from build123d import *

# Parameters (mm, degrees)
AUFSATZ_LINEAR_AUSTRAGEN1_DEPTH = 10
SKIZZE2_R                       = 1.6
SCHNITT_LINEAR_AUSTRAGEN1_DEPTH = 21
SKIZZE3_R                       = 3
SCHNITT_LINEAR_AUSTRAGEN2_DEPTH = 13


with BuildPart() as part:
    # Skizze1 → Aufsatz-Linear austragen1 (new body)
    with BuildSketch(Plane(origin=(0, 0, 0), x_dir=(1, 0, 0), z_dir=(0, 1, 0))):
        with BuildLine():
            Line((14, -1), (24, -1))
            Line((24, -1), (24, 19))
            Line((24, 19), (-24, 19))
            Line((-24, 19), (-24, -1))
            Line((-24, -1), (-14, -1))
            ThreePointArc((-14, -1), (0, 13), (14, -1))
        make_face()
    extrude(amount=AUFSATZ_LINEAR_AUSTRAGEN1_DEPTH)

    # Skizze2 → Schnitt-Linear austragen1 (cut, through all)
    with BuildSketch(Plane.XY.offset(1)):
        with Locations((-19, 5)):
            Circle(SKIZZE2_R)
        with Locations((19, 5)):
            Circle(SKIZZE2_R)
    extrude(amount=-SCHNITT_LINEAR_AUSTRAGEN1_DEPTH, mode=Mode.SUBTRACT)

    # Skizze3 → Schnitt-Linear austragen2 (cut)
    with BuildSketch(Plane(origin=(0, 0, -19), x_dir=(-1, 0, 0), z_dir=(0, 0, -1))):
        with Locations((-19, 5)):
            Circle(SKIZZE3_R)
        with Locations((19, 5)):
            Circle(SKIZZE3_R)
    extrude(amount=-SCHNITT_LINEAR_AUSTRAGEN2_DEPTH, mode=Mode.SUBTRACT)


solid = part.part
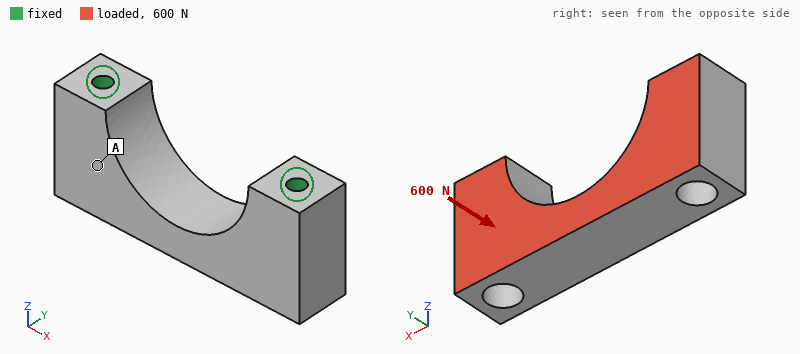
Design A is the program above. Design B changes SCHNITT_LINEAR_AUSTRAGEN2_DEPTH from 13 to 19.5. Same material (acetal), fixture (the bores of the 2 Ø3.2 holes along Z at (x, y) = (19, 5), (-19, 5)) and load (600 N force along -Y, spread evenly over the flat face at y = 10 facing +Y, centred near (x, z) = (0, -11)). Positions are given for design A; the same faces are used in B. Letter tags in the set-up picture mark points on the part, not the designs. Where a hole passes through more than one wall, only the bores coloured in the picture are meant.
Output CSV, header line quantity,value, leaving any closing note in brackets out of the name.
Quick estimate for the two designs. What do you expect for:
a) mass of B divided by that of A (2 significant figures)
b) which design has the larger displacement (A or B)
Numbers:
quantity,value
mass of B divided by that of A,0.95
which design has the larger displacement,B
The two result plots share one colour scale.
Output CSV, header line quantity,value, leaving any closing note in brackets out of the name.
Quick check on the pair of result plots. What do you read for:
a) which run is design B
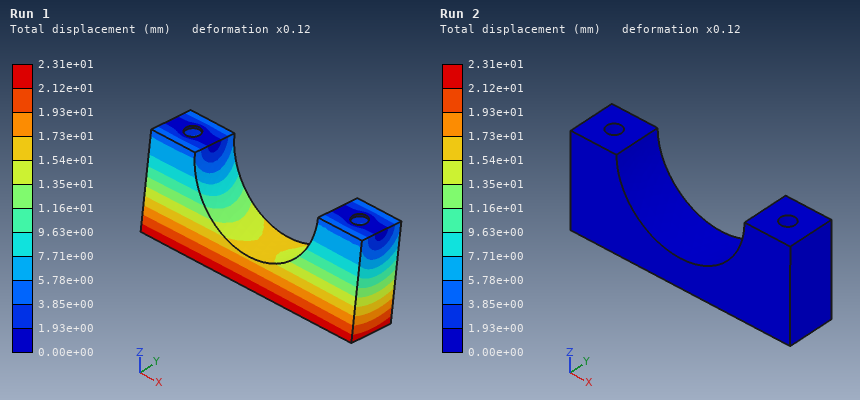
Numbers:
quantity,value
which run is design B,Run 1
